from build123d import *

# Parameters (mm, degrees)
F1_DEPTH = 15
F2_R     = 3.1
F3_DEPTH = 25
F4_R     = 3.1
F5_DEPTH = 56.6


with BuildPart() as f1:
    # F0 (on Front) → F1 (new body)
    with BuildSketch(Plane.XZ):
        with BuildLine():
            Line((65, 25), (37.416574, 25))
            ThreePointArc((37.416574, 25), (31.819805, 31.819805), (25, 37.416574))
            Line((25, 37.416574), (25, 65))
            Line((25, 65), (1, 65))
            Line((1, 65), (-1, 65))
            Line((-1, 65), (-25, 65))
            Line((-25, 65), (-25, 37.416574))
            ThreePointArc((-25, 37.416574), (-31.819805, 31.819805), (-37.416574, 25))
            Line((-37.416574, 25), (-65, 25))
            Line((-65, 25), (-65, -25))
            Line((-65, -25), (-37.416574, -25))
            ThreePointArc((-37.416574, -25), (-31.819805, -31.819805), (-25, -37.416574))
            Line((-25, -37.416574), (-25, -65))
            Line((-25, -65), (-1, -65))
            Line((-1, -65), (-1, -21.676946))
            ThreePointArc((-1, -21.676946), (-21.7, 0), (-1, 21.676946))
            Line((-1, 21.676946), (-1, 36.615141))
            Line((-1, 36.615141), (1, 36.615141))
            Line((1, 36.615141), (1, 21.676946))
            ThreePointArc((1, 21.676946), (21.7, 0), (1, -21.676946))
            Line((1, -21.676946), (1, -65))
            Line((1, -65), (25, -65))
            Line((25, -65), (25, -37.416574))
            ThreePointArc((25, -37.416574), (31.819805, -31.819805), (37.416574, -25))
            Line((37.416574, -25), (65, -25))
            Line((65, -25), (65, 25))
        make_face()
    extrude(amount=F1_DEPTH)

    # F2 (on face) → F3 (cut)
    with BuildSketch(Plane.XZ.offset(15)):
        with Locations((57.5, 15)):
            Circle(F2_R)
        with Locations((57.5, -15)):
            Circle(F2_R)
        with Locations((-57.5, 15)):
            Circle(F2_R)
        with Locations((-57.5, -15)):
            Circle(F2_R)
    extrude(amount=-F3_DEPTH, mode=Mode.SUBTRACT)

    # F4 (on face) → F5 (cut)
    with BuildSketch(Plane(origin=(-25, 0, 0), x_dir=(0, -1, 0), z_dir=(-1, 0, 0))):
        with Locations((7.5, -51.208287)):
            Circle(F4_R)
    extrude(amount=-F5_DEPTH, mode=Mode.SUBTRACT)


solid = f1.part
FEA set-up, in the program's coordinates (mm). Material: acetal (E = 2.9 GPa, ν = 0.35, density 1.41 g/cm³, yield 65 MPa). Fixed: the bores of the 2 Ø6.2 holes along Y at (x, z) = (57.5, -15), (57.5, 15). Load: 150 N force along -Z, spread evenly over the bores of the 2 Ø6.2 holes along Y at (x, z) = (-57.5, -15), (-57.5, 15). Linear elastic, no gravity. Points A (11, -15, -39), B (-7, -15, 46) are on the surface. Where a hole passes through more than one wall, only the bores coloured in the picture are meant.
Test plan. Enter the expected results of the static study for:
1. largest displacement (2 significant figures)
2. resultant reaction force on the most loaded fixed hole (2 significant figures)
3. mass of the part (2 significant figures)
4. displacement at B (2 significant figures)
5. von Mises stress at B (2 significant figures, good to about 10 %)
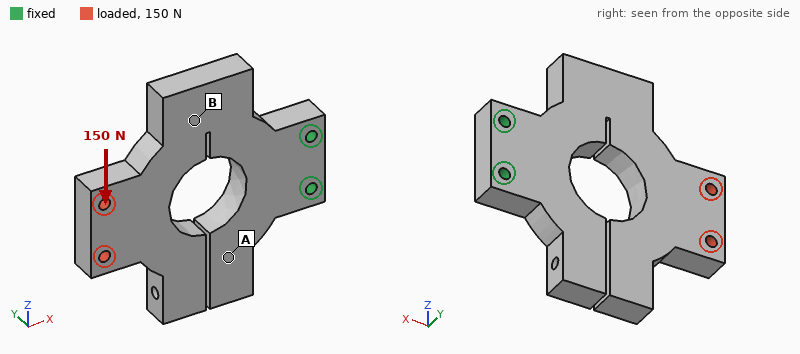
1.9 mm
550 N
190 g
0.46 mm
2.9 MPa
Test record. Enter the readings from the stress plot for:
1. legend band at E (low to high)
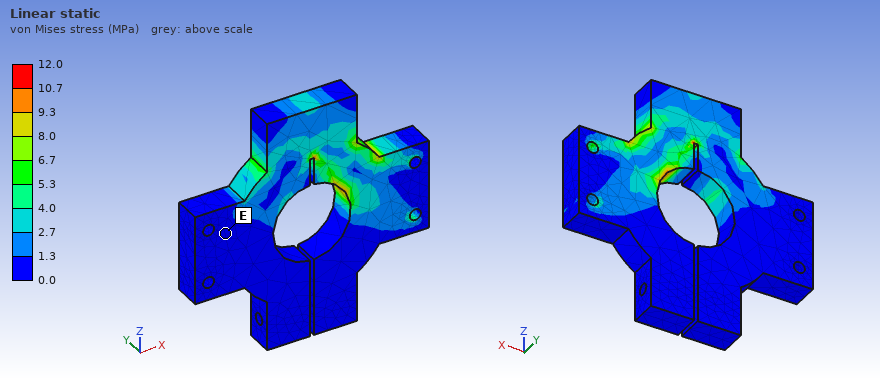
0.0 to 1.3 MPa
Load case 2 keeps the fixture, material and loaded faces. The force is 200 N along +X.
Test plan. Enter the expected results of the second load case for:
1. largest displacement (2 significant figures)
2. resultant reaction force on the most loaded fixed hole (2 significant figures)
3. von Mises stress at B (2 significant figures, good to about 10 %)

1.3 mm
110 N
2.7 MPa
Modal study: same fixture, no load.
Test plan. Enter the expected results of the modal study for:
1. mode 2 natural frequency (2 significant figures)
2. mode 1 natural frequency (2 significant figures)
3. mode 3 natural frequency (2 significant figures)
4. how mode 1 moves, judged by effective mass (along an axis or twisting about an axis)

200 Hz
120 Hz
240 Hz
along Y
